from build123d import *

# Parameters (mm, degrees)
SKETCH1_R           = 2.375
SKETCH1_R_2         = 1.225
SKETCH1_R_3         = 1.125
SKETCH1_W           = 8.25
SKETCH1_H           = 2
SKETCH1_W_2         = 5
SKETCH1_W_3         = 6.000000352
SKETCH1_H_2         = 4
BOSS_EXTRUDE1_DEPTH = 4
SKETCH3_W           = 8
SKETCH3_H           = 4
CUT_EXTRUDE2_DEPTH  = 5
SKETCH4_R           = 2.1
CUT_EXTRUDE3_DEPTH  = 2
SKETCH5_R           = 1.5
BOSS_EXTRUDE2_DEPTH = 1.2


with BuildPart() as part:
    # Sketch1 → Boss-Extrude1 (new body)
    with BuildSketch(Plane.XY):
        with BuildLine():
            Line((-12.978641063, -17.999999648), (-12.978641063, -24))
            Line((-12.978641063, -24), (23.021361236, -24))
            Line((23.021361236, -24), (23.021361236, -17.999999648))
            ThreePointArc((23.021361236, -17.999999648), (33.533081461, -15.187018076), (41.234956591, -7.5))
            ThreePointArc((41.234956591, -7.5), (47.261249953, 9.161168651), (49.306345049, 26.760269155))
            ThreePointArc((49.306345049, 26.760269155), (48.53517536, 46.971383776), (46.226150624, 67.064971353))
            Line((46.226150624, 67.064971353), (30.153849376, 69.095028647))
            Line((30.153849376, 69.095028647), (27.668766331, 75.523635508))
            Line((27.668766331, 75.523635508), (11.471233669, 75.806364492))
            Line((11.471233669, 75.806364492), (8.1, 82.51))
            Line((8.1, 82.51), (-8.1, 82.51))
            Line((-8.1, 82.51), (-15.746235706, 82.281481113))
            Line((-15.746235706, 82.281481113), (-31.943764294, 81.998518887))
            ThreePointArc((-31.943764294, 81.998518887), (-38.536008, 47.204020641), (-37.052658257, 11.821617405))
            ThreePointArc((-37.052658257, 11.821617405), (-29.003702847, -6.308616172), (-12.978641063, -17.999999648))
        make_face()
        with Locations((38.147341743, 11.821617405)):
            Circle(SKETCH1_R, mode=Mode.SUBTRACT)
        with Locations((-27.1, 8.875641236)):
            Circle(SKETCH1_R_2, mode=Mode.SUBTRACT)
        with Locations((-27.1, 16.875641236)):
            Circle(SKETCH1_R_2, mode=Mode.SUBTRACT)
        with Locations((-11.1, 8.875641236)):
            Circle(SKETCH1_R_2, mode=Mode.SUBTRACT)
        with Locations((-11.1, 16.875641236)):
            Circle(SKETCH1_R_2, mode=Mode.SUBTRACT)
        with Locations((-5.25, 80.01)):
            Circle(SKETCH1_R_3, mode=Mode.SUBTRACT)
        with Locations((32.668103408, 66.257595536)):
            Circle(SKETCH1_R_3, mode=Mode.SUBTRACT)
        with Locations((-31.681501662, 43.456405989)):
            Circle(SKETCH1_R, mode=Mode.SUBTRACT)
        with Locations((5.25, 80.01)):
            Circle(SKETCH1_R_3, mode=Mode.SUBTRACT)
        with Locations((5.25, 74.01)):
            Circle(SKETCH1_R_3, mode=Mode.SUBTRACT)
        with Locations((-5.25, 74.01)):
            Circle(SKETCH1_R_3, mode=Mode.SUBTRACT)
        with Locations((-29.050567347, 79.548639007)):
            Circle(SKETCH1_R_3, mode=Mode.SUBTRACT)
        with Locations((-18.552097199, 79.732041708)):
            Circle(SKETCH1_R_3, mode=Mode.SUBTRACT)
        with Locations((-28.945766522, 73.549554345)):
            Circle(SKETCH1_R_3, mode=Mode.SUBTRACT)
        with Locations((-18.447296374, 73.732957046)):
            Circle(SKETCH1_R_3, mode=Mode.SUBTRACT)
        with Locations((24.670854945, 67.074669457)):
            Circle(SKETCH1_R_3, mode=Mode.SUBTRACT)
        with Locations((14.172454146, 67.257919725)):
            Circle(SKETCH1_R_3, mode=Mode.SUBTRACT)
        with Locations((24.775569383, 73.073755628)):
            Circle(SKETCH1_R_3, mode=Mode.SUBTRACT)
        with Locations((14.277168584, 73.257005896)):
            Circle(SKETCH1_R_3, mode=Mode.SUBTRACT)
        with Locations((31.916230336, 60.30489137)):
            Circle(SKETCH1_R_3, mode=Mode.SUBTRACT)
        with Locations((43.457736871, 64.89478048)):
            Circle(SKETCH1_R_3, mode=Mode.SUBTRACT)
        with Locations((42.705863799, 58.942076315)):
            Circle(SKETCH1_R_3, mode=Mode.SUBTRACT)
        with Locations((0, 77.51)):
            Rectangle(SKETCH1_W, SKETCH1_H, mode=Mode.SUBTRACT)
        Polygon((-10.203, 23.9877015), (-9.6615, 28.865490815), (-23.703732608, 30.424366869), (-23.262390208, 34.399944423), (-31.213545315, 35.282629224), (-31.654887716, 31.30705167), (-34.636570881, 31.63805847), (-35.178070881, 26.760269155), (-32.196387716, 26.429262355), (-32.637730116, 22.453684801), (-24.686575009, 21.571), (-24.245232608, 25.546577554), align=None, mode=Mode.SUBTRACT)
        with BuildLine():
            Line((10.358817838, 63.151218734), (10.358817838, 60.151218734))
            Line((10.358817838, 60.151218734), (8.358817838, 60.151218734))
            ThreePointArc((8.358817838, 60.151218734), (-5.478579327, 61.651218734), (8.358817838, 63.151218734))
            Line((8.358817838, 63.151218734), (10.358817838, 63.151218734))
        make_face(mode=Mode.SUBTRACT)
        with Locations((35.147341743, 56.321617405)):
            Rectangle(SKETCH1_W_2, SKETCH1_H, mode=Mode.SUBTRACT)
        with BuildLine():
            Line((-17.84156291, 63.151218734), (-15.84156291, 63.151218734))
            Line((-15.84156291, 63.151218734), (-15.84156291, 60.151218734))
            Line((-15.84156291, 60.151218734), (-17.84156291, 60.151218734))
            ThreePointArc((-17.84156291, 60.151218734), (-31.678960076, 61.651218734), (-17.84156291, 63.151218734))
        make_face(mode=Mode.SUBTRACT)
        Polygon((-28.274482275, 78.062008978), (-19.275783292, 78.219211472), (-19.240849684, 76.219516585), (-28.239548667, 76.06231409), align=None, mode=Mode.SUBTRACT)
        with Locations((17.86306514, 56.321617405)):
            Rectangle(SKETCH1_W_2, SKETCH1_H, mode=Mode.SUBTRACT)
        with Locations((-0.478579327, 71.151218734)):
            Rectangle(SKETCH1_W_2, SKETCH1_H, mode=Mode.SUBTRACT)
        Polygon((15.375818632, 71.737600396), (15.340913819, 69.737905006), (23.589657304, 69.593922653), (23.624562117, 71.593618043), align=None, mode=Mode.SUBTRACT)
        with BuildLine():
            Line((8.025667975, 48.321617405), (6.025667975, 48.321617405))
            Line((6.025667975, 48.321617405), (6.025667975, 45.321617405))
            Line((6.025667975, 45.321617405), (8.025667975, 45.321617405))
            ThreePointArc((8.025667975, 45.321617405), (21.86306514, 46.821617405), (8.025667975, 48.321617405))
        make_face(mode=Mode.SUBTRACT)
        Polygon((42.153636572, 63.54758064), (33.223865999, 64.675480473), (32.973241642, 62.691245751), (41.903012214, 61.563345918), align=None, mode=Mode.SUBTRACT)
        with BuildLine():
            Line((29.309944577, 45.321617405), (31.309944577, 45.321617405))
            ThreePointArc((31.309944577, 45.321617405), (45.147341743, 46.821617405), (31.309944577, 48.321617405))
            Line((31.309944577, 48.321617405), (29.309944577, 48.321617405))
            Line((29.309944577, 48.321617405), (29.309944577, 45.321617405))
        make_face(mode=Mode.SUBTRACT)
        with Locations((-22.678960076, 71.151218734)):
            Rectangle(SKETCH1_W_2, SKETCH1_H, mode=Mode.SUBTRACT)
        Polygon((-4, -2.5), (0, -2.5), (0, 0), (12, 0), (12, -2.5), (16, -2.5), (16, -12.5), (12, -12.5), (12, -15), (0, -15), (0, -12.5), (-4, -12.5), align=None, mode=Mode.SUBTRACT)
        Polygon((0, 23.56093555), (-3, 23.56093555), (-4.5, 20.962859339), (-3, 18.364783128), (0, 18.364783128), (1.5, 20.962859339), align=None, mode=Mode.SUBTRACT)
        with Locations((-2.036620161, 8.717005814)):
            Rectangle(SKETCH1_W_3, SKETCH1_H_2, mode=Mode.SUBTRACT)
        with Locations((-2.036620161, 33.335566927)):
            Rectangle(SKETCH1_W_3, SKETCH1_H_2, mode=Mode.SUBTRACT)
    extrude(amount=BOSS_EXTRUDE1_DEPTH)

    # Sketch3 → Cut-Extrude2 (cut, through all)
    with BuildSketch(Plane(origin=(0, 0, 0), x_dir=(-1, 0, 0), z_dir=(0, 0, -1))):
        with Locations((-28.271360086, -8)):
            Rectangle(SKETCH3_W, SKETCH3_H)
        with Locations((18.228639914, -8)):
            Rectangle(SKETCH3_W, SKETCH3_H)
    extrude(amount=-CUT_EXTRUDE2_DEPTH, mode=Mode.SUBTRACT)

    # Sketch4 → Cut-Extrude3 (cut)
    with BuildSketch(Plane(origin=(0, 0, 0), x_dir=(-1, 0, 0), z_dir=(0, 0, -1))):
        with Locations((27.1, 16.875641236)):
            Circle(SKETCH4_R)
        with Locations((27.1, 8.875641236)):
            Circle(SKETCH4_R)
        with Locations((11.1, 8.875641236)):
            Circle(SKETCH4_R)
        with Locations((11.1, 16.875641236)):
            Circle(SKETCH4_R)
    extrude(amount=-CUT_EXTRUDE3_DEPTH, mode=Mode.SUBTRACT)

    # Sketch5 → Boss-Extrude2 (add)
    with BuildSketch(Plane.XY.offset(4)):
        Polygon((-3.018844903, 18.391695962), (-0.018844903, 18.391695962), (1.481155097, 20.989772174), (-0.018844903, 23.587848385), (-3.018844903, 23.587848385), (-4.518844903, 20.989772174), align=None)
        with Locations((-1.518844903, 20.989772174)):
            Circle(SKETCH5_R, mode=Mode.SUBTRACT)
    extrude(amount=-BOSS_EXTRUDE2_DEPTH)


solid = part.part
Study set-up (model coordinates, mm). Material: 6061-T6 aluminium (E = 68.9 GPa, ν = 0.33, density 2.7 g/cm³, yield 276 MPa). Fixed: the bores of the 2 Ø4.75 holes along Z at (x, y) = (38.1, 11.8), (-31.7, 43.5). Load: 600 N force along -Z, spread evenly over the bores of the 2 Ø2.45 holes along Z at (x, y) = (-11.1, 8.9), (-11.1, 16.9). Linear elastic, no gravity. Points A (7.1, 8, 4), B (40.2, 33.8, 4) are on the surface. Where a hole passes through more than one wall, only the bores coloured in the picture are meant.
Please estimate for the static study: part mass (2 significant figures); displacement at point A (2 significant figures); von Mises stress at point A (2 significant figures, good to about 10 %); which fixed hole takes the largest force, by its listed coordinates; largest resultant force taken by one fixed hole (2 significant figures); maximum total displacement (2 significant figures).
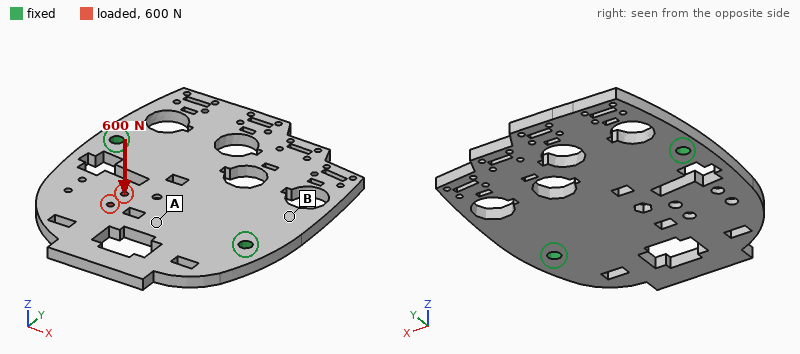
70 g
0.19 mm
28 MPa
(-31.7, 43.5)
340 N
0.55 mm
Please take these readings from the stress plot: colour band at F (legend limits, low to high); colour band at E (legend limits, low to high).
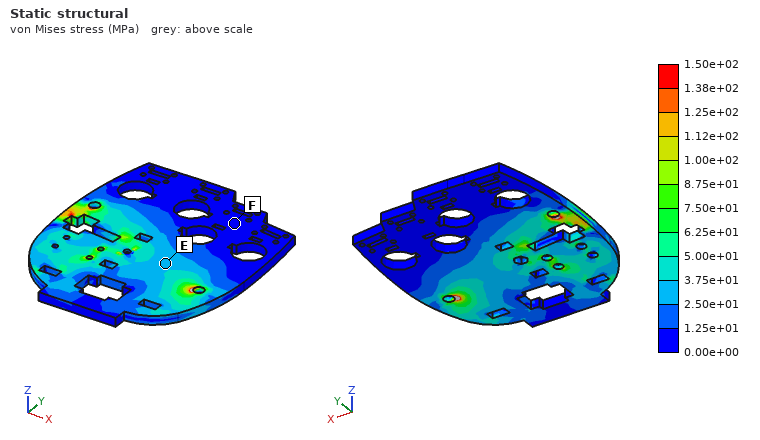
0.00e+00 to 1.25e+01 MPa
2.50e+01 to 3.75e+01 MPa
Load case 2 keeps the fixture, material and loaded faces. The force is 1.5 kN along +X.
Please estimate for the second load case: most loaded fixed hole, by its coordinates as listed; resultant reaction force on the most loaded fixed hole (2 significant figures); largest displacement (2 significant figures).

(38.1, 11.8)
1.1 kN
39 µm
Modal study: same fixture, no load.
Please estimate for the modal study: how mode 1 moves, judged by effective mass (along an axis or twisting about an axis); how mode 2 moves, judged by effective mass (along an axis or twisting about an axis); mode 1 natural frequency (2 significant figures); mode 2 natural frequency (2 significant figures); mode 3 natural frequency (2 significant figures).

twisting about X
along Z
1000 Hz
1400 Hz
2400 Hz
